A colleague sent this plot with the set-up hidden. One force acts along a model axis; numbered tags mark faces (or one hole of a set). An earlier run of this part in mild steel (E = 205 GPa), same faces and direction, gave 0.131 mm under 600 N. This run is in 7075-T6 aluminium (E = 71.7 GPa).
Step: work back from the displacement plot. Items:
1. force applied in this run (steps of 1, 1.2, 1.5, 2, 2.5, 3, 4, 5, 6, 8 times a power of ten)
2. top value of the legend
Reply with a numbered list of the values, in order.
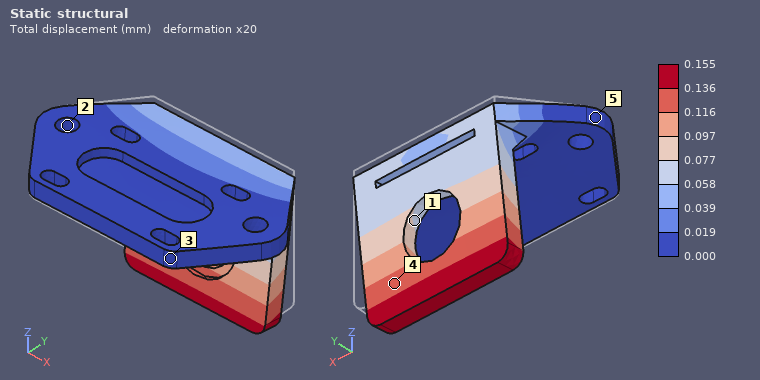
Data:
1. 250 N
2. 0.155 mm
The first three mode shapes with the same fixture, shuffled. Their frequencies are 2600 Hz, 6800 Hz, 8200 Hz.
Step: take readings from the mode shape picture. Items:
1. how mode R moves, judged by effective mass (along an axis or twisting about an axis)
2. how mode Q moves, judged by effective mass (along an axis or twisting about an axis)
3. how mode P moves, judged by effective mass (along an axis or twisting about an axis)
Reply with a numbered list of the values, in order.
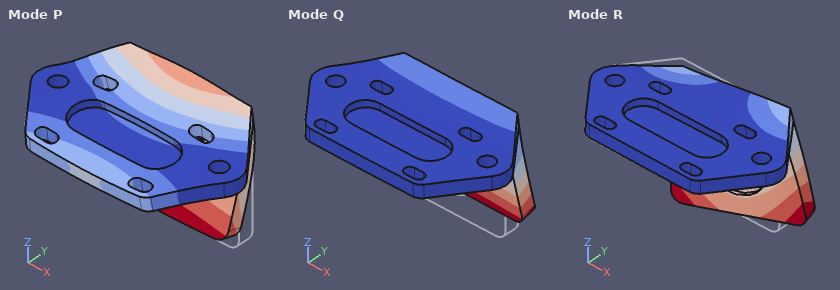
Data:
1. along X
2. along Y
3. along Z
